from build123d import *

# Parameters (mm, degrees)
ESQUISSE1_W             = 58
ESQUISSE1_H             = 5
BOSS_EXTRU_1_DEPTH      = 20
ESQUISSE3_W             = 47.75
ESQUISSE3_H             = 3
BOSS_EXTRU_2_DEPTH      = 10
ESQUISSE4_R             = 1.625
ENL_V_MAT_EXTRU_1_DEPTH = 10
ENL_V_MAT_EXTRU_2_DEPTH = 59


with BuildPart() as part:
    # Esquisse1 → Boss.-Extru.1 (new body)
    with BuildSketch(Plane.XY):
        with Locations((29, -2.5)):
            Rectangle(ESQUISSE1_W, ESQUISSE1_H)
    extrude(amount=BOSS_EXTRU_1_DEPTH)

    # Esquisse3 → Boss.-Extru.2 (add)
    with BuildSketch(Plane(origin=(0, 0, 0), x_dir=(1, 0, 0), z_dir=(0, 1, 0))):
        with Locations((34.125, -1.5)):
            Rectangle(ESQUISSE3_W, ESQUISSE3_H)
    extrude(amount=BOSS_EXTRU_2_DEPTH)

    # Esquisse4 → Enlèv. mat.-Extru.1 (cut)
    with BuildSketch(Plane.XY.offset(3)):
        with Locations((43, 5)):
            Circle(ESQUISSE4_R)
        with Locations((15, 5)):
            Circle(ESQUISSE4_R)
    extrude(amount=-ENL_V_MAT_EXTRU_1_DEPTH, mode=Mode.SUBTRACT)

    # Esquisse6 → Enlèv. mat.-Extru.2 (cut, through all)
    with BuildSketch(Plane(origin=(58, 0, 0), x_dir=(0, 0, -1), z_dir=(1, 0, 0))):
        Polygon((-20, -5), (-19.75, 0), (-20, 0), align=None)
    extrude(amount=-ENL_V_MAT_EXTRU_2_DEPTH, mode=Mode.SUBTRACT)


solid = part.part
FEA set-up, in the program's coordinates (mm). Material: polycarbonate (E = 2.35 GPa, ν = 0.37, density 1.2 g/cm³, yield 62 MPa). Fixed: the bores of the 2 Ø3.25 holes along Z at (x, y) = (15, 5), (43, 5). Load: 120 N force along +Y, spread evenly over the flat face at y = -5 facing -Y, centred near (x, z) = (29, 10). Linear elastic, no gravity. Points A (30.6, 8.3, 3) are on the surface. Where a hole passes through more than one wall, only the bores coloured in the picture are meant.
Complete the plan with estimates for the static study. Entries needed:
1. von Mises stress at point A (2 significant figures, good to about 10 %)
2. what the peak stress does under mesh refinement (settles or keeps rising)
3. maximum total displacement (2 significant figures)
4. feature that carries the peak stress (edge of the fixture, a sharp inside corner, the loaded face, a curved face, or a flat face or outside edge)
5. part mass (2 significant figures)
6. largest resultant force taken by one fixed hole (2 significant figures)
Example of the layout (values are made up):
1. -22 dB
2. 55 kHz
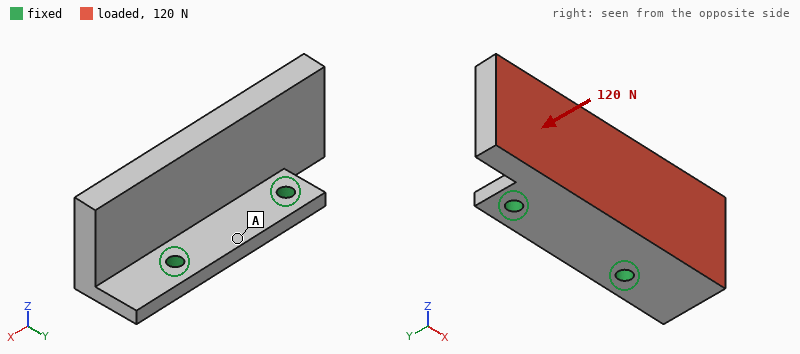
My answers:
1. 4.1 MPa
2. keeps rising
3. 0.75 mm
4. edge of the fixture
5. 8.6 g
6. 61 N
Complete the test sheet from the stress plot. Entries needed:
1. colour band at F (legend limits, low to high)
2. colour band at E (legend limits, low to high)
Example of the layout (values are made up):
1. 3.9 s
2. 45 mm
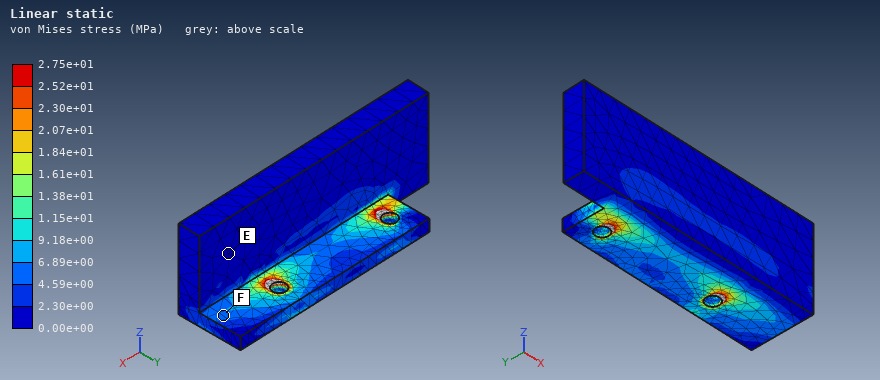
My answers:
1. 4.59e+00 to 6.89e+00 MPa
2. 0.00e+00 to 2.30e+00 MPa
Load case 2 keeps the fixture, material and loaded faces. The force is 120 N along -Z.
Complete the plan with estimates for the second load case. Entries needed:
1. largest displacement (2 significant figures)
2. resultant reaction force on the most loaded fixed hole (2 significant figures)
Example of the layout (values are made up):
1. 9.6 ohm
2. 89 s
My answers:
1. 0.58 mm
2. 60 N
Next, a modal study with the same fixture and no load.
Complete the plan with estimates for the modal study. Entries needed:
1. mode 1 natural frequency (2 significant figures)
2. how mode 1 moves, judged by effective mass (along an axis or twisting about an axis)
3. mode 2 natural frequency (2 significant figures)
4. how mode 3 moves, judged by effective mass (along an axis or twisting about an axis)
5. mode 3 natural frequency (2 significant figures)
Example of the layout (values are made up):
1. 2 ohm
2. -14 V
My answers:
1. 930 Hz
2. along Y
3. 1700 Hz
4. along X
5. 2800 Hz
